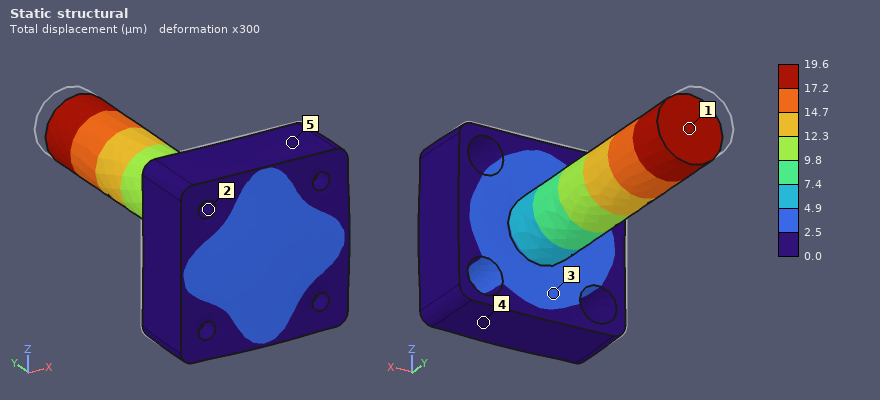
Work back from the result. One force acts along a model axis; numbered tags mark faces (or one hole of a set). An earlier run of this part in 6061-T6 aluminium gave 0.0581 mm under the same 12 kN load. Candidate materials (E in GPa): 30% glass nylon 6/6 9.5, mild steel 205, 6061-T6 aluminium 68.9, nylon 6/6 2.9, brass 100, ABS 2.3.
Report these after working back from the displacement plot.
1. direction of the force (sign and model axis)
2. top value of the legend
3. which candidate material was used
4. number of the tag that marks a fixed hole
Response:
-Y
19.6 µm
mild steel
2
